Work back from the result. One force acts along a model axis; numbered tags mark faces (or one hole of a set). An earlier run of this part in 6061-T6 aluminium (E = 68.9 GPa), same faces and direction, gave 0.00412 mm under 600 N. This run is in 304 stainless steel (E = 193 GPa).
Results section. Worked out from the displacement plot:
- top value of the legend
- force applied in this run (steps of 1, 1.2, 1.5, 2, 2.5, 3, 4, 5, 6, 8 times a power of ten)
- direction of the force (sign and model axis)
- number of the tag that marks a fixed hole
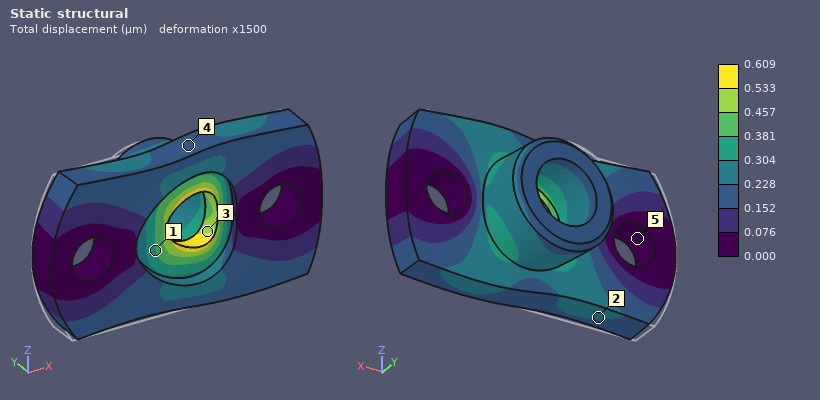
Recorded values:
0.609 µm
250 N
+X
5
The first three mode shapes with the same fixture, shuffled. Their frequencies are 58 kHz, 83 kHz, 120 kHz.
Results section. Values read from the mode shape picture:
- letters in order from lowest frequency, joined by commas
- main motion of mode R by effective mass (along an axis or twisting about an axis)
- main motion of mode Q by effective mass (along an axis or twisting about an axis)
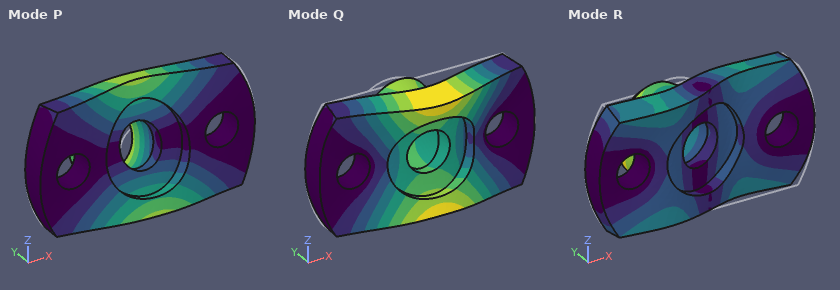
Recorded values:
P, Q, R
along X
along Y
